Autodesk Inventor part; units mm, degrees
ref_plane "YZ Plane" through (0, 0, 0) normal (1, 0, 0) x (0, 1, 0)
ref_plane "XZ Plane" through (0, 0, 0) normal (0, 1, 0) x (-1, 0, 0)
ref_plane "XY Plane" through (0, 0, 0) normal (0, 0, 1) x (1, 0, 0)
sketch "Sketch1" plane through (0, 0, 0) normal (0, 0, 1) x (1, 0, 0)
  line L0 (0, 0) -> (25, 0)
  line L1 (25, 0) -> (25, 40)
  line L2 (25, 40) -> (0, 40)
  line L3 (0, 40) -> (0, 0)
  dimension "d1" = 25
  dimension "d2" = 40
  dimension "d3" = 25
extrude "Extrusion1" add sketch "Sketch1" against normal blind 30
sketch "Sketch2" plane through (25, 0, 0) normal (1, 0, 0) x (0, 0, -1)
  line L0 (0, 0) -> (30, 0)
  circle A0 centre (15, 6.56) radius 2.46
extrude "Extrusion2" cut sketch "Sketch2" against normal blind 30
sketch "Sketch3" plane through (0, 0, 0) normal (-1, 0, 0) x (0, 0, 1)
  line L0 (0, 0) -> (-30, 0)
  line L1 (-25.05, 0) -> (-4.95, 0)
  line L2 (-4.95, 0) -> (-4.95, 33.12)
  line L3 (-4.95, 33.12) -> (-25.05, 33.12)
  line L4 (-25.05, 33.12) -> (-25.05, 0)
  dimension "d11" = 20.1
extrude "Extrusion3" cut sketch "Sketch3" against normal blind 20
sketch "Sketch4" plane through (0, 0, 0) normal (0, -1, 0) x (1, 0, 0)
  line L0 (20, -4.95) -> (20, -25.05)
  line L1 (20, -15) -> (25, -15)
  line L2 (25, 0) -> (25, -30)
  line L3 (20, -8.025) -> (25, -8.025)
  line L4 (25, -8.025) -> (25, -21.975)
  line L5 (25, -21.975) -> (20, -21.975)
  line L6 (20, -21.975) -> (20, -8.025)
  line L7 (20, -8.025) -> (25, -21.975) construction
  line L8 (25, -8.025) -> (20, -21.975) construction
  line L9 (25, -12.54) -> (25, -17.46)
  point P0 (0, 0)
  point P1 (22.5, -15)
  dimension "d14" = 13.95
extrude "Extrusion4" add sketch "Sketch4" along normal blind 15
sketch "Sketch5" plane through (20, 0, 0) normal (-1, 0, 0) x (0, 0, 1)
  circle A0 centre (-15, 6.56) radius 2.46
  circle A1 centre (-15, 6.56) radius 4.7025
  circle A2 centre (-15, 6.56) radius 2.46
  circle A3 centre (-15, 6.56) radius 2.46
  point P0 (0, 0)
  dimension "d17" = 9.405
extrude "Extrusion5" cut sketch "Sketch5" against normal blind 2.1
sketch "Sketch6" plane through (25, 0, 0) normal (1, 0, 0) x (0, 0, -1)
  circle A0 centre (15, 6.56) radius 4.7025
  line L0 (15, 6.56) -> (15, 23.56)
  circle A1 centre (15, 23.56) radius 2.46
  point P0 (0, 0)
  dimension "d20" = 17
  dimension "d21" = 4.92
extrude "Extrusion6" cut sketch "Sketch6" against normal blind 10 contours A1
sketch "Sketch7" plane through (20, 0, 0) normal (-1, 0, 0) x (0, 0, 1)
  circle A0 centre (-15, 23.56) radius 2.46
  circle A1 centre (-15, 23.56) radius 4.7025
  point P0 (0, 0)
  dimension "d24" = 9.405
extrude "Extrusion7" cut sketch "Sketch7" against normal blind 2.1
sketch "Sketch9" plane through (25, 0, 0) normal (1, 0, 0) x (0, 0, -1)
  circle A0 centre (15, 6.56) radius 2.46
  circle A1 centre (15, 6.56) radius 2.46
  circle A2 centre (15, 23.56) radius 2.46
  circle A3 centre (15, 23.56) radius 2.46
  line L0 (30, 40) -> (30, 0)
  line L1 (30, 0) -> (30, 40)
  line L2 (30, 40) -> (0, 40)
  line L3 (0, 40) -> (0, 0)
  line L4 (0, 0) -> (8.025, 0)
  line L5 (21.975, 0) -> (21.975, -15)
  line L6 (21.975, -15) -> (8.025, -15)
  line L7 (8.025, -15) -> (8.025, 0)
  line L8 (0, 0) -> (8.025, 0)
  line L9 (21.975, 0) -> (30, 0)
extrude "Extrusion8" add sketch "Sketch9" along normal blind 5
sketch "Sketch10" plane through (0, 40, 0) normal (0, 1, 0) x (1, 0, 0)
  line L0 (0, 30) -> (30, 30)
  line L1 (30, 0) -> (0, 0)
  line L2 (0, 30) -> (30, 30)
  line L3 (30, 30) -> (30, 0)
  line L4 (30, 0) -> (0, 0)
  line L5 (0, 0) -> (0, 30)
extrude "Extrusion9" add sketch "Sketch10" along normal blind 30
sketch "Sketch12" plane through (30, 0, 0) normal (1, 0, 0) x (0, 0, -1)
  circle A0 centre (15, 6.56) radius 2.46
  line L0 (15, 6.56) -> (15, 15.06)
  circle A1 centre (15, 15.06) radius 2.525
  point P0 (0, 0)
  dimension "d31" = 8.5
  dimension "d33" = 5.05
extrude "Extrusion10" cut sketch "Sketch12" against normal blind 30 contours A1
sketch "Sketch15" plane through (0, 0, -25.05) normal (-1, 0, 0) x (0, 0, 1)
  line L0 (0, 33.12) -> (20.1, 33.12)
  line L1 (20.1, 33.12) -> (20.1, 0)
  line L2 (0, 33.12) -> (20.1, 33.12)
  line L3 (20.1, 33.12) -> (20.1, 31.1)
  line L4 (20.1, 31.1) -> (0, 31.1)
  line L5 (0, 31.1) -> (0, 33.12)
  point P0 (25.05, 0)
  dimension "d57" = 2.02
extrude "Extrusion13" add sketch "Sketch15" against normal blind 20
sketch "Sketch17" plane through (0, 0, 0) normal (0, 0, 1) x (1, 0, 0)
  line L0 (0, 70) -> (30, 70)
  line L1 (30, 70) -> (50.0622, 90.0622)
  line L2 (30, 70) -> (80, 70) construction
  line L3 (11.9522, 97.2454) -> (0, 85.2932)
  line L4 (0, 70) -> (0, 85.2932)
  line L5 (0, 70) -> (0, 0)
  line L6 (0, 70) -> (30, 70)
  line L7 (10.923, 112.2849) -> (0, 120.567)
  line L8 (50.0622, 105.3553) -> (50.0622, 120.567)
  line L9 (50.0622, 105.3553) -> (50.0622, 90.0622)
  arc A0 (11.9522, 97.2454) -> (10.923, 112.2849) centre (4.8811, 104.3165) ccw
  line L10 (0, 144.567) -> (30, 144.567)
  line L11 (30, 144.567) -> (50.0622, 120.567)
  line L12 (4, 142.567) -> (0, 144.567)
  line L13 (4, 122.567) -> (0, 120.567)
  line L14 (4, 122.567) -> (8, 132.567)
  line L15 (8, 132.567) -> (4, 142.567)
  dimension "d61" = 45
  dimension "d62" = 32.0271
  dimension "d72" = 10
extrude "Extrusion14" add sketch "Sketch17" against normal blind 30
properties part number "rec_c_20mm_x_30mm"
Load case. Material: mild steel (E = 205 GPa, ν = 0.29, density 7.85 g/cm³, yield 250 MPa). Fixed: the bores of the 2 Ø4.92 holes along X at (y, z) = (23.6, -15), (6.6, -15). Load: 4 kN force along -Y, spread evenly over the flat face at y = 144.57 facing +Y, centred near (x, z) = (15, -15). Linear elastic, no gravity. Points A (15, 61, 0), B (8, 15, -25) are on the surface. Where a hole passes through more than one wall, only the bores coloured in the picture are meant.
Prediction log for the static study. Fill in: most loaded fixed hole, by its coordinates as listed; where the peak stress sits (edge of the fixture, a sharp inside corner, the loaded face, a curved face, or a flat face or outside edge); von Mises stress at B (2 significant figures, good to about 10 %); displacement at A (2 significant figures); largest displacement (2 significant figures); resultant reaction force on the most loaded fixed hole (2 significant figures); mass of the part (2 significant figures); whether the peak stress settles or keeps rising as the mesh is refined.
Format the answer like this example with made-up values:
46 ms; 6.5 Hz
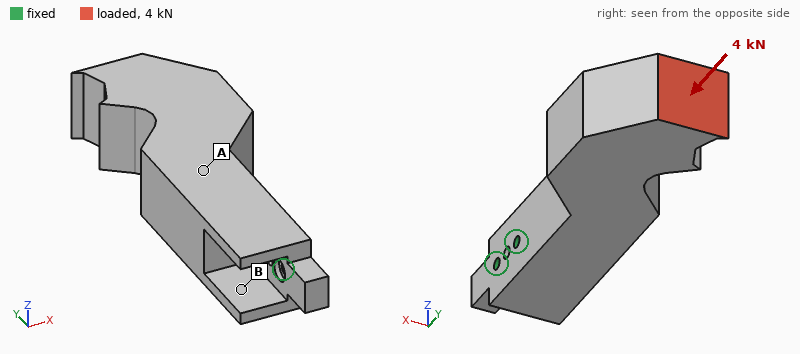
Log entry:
(23.6, -15); edge of the fixture; 11 MPa; 12 µm; 49 µm; 3.0 kN; 1.1 kg; keeps rising
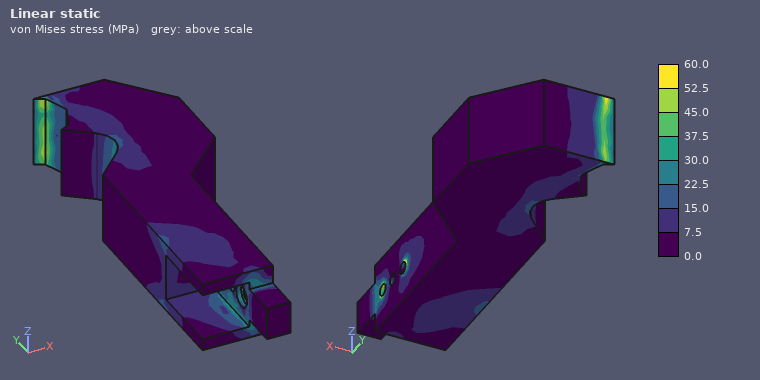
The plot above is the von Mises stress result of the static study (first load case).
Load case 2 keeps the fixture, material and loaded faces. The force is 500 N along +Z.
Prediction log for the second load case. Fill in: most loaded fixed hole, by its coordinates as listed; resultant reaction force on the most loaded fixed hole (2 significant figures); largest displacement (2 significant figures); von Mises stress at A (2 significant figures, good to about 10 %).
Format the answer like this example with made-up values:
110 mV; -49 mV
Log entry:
(23.6, -15); 3.1 kN; 57 µm; 9.0 MPa
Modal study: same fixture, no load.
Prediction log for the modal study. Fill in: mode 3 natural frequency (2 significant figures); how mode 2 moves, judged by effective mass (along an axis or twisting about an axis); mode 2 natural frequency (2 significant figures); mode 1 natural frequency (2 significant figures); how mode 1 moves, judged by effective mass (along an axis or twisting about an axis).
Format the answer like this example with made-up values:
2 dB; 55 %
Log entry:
2400 Hz; along Z; 840 Hz; 720 Hz; along X
